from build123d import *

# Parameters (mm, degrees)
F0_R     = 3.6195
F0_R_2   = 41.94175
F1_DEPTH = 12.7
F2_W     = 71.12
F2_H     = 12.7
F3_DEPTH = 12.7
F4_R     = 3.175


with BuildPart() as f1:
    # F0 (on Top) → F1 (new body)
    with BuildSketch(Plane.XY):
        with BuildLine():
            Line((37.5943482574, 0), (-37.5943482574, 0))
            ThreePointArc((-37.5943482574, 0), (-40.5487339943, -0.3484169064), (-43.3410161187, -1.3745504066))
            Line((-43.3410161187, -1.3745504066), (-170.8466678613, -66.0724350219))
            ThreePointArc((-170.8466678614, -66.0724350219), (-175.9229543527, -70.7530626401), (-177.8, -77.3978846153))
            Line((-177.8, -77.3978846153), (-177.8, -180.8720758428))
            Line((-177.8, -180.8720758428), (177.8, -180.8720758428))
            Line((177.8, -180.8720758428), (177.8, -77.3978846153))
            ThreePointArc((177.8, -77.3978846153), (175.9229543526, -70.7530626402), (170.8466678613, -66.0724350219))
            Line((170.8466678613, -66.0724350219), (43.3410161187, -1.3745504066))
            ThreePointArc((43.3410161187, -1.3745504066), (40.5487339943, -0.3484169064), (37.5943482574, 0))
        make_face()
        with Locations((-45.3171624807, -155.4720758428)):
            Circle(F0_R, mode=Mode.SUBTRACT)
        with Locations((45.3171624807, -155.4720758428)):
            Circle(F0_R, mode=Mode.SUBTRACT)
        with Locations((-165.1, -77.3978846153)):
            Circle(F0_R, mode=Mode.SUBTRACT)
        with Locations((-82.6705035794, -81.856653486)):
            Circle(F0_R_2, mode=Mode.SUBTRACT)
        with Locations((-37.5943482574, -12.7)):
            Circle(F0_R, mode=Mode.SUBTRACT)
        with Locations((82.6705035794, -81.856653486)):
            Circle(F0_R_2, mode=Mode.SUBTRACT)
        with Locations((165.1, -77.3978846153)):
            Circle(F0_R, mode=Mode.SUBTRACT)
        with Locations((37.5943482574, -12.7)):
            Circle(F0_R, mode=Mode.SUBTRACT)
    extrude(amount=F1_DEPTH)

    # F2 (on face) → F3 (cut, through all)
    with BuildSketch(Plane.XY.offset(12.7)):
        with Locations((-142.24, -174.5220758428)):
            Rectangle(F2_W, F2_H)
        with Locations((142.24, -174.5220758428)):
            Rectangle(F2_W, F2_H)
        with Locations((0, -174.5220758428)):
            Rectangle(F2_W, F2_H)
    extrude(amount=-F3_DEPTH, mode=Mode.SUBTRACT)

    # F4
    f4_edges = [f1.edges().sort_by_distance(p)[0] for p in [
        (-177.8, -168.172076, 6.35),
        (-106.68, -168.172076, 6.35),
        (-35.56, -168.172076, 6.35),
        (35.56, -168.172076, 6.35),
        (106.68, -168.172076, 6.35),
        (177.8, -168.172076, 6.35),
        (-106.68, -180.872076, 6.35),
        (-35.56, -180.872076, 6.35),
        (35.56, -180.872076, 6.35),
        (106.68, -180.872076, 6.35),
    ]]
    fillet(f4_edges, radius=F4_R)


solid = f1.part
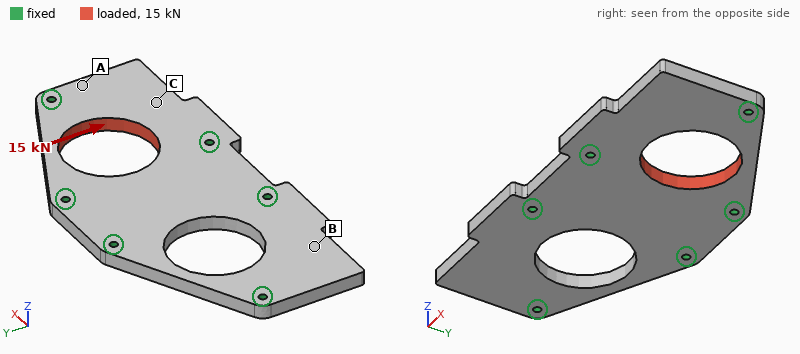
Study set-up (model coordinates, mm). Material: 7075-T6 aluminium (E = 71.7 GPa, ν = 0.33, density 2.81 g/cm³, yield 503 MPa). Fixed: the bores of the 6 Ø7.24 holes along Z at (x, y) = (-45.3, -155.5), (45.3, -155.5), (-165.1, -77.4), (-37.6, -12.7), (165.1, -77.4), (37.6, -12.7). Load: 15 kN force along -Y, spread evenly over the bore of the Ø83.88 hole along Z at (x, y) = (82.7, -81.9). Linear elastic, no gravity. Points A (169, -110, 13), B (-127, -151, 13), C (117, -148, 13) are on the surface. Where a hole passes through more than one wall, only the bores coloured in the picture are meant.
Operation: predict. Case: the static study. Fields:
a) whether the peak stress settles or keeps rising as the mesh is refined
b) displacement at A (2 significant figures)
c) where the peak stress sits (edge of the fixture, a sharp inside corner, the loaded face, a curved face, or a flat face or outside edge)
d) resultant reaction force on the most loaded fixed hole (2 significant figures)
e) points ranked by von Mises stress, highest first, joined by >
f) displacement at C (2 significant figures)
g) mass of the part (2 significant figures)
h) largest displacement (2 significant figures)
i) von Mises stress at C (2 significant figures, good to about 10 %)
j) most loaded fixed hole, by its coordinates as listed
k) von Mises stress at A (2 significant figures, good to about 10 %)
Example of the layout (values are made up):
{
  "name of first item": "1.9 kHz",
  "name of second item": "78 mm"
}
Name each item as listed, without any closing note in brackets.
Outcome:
{
  "whether the peak stress settles or keeps rising as the mesh is refined": "keeps rising",
  "displacement at A": "7.1 µm",
  "where the peak stress sits": "edge of the fixture",
  "resultant reaction force on the most loaded fixed hole": "5.7 kN",
  "points ranked by von Mises stress, highest first, joined by >": "A > C > B",
  "displacement at C": "14 µm",
  "mass of the part": "1.5 kg",
  "largest displacement": "36 µm",
  "von Mises stress at C": "5.6 MPa",
  "most loaded fixed hole, by its coordinates as listed": "(165.1, -77.4)",
  "von Mises stress at A": "9.3 MPa"
}
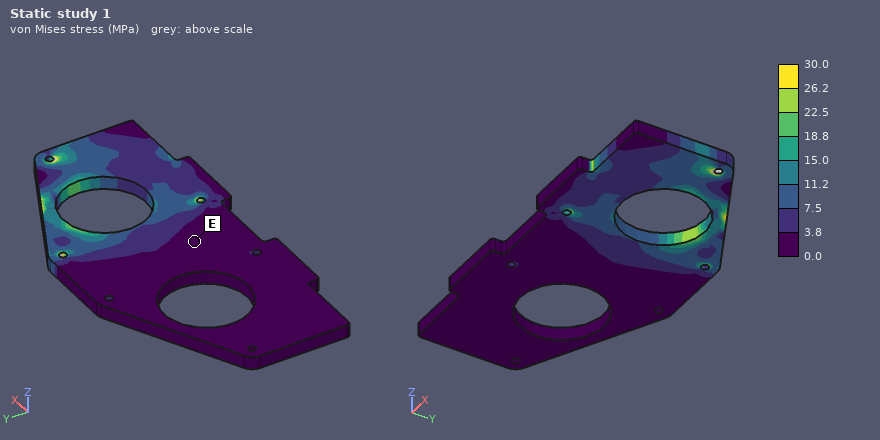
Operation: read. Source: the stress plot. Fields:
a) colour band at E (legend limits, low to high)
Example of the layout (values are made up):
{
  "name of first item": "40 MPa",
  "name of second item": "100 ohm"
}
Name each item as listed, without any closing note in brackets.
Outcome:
{
  "colour band at E": "0.0 to 3.8 MPa"
}
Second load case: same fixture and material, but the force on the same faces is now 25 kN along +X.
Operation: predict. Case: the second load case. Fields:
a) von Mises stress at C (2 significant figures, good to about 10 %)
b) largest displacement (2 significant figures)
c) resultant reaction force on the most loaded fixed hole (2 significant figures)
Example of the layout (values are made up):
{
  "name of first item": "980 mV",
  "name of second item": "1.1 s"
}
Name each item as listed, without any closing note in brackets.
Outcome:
{
  "von Mises stress at C": "4.4 MPa",
  "largest displacement": "27 µm",
  "resultant reaction force on the most loaded fixed hole": "6.7 kN"
}
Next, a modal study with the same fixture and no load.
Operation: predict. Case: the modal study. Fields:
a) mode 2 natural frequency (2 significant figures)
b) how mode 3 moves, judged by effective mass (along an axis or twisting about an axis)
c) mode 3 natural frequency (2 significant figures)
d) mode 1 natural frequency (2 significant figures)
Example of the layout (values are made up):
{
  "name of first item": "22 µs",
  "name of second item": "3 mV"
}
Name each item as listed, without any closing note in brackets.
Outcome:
{
  "mode 2 natural frequency": "1600 Hz",
  "how mode 3 moves, judged by effective mass": "along Z",
  "mode 3 natural frequency": "2800 Hz",
  "mode 1 natural frequency": "1600 Hz"
}
